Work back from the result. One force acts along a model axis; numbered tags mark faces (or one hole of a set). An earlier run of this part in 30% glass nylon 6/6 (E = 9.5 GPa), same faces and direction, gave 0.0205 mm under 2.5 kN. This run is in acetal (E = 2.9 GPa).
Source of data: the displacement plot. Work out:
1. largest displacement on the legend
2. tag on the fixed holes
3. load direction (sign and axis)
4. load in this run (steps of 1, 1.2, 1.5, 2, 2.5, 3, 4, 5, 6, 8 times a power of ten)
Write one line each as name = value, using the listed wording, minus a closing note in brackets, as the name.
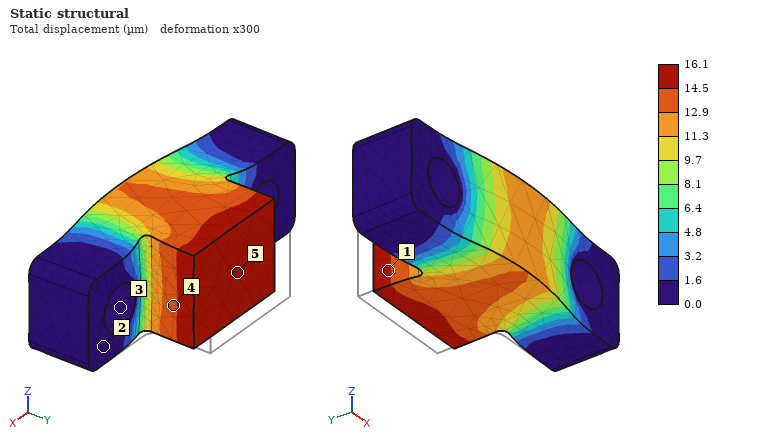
largest displacement on the legend = 16.1 µm
tag on the fixed holes = 3
load direction = -Y
load in this run = 600 N
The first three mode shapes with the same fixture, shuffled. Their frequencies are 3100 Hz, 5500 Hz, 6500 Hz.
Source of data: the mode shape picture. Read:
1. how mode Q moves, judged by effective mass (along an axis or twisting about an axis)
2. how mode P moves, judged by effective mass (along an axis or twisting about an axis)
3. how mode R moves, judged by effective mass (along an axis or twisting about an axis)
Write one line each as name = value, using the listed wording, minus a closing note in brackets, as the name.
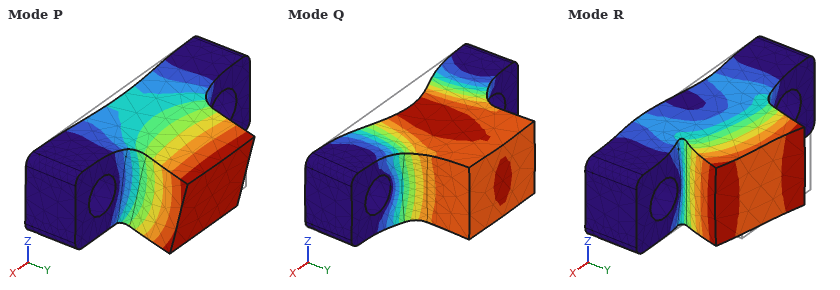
how mode Q moves, judged by effective mass = along Y
how mode P moves, judged by effective mass = along Z
how mode R moves, judged by effective mass = along X
